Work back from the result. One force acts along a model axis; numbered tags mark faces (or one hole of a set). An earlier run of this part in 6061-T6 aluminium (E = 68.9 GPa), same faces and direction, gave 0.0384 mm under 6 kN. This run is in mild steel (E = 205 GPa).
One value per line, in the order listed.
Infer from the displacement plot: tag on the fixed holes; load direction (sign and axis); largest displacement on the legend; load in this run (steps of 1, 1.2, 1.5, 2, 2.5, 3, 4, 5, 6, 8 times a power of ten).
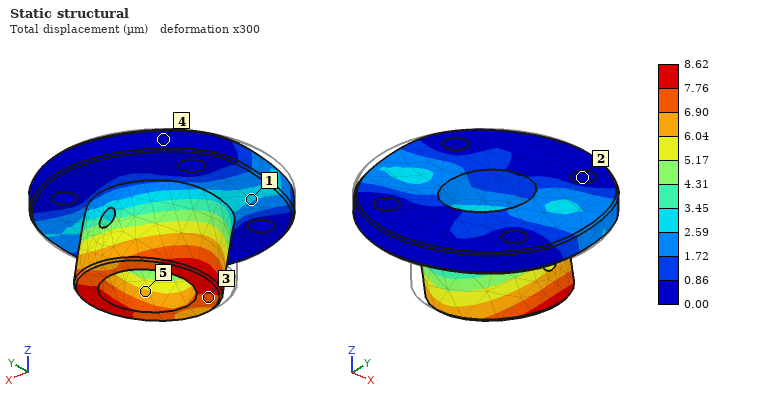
2
+X
8.62 µm
4 kN
